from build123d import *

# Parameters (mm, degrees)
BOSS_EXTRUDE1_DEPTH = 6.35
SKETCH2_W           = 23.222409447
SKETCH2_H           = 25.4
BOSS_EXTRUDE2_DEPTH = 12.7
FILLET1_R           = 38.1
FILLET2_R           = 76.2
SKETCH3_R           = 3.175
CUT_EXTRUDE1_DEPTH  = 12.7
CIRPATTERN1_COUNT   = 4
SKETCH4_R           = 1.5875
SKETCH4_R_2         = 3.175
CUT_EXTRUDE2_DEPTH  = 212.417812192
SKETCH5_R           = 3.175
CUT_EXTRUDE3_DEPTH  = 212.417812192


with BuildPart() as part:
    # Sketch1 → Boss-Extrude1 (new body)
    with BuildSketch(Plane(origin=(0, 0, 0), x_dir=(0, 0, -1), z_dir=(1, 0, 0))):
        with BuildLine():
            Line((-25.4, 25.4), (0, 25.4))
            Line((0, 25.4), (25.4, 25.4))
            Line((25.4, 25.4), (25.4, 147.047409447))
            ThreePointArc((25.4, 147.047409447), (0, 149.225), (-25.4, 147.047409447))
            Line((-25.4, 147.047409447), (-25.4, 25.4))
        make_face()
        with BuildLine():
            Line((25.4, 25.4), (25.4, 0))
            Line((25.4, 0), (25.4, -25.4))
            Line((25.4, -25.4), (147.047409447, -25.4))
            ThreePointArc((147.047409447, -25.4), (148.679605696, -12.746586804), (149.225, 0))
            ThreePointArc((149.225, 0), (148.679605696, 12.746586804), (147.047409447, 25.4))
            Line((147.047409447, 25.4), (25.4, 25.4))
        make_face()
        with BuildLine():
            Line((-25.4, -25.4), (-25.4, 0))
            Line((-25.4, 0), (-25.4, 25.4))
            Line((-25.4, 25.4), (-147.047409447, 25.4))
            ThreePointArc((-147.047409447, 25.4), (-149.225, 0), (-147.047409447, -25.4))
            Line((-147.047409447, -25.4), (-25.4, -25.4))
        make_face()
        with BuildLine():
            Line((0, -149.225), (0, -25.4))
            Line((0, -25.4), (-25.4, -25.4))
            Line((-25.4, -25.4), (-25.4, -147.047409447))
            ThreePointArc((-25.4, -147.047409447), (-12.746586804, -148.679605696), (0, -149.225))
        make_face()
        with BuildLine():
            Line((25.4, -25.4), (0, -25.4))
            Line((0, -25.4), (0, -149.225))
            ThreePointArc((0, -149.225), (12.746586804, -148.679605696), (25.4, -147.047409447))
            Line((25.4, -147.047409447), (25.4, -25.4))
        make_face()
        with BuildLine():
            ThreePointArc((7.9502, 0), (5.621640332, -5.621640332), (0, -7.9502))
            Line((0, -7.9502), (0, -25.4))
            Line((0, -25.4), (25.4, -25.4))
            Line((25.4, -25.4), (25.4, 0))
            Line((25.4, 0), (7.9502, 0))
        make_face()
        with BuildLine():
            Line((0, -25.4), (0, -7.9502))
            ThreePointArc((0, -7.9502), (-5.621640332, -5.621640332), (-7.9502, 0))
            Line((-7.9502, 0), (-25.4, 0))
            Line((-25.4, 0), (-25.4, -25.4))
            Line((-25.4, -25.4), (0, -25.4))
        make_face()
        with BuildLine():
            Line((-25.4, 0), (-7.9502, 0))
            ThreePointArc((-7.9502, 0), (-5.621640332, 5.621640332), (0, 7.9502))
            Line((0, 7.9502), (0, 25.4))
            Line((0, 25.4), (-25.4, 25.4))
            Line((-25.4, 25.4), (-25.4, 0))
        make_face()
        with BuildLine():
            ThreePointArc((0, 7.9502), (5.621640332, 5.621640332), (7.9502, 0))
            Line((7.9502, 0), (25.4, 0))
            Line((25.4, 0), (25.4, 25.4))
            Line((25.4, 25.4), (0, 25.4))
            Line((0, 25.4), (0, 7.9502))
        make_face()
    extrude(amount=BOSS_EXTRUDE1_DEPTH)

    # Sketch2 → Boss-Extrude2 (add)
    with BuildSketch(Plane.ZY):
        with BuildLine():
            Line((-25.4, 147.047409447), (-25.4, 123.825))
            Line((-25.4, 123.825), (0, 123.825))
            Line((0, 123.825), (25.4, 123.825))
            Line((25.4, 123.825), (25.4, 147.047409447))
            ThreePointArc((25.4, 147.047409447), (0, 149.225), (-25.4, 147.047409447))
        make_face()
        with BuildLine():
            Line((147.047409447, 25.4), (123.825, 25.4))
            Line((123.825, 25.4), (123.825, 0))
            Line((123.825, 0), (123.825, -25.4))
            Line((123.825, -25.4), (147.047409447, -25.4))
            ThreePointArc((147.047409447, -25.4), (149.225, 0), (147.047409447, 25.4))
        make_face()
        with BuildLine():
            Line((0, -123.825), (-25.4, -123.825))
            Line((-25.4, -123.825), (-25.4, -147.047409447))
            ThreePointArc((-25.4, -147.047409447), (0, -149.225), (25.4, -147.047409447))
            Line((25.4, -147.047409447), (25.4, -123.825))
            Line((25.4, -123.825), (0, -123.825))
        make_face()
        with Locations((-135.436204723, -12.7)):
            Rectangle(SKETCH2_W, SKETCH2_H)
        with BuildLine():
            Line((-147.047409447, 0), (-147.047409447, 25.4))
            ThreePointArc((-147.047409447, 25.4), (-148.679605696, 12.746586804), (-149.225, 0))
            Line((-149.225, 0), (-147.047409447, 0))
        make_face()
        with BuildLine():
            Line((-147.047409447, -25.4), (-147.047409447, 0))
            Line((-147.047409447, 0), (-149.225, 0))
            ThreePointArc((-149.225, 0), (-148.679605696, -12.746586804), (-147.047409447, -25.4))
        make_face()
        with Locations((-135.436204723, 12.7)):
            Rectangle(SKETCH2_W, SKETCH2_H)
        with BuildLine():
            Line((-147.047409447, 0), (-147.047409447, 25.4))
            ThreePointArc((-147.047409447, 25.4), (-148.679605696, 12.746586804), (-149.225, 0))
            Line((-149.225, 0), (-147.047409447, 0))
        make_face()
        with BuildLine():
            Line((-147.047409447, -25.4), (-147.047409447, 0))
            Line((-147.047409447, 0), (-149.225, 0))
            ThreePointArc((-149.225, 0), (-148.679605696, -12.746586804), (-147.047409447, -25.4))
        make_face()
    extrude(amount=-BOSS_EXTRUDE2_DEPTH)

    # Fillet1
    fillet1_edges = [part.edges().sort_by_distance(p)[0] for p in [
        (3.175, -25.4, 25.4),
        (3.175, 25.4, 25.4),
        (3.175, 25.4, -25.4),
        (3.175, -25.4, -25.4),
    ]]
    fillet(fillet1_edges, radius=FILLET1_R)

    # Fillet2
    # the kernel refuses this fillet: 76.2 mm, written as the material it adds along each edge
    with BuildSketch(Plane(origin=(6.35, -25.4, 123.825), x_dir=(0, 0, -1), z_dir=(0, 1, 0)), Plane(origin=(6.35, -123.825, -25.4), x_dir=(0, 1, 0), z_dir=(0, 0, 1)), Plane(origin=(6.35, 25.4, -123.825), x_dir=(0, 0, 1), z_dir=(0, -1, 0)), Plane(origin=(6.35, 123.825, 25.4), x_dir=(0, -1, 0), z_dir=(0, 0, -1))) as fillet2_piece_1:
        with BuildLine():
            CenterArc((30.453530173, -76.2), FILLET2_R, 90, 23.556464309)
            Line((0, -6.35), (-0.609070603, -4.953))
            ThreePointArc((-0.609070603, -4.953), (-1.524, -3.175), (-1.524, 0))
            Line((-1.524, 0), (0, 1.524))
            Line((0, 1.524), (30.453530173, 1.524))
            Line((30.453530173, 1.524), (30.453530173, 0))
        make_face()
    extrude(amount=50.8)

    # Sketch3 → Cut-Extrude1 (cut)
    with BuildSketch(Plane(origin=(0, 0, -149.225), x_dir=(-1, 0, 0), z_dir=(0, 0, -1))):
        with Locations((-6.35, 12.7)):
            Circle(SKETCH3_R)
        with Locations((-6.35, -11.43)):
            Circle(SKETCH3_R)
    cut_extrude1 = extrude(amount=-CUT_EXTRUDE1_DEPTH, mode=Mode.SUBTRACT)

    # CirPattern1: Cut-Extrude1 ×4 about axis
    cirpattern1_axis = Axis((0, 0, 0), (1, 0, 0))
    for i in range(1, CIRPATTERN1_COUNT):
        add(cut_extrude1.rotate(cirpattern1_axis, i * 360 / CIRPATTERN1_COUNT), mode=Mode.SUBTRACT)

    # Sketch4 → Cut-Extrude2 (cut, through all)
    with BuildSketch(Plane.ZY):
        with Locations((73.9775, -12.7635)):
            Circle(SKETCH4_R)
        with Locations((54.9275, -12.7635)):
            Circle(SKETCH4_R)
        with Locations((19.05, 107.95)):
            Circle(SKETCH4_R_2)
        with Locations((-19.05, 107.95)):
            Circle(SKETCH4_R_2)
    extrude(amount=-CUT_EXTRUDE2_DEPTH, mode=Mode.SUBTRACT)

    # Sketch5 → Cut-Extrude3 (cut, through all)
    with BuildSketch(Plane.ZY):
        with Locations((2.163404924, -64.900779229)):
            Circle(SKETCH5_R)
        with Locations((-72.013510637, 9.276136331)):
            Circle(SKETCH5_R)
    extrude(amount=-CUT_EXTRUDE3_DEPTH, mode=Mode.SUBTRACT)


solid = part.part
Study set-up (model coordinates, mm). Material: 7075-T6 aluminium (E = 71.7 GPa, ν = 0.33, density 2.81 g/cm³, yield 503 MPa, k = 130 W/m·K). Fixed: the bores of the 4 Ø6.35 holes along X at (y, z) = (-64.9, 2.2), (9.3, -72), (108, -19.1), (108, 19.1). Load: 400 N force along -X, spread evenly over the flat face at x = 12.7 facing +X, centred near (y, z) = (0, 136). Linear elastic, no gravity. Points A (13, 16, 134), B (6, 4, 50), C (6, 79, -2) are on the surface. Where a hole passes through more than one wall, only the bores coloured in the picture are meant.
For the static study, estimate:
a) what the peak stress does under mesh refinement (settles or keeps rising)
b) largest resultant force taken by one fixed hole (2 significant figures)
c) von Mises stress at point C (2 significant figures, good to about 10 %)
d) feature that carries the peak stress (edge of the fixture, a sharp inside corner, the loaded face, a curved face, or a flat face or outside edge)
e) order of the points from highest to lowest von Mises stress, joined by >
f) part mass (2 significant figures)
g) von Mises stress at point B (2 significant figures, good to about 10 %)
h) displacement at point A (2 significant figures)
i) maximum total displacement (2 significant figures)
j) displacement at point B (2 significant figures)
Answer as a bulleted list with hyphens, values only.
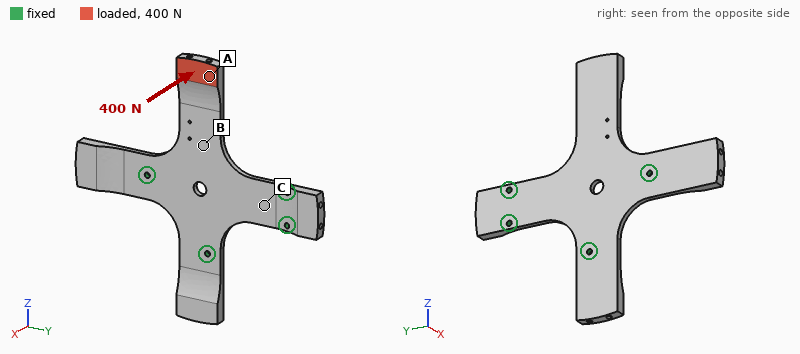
- keeps rising
- 490 N
- 32 MPa
- edge of the fixture
- B > C > A
- 630 g
- 95 MPa
- 3.8 mm
- 4.4 mm
- 0.84 mm
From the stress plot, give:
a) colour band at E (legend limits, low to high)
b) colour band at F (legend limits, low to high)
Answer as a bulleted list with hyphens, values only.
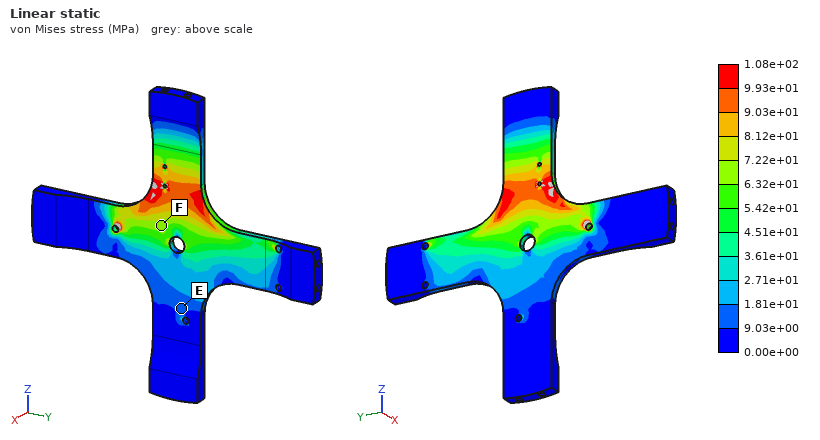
- 9.03e+00 to 1.81e+01 MPa
- 6.32e+01 to 7.22e+01 MPa
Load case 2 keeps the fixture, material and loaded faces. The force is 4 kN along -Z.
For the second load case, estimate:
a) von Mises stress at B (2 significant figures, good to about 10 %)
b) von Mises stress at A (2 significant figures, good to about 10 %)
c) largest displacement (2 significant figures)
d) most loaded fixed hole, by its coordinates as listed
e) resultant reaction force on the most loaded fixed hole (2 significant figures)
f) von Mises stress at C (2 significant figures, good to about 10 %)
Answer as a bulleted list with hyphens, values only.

- 110 MPa
- 17 MPa
- 4.5 mm
- (9.3, -72)
- 2.2 kN
- 26 MPa
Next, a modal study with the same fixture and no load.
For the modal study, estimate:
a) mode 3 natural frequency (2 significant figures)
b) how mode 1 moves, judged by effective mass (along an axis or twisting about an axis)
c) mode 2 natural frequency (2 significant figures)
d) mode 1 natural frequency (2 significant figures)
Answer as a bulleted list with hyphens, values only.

- 640 Hz
- along X
- 550 Hz
- 190 Hz
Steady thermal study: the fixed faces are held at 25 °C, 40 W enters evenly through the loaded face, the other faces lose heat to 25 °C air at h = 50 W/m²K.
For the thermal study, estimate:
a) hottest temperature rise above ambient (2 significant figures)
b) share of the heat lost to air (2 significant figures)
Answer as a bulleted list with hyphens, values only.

- 58 K
- 75 %
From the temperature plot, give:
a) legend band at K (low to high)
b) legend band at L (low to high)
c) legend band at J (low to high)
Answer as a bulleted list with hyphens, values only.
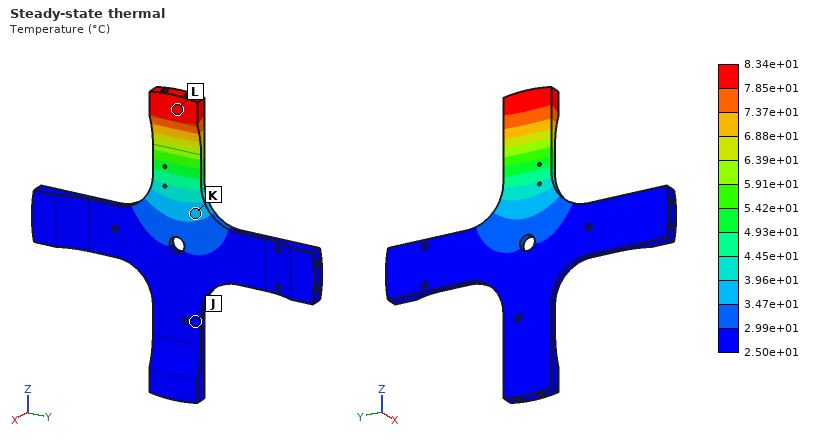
- 3.47e+01 to 3.96e+01 °C
- 7.85e+01 to 8.34e+01 °C
- 2.50e+01 to 2.99e+01 °C
